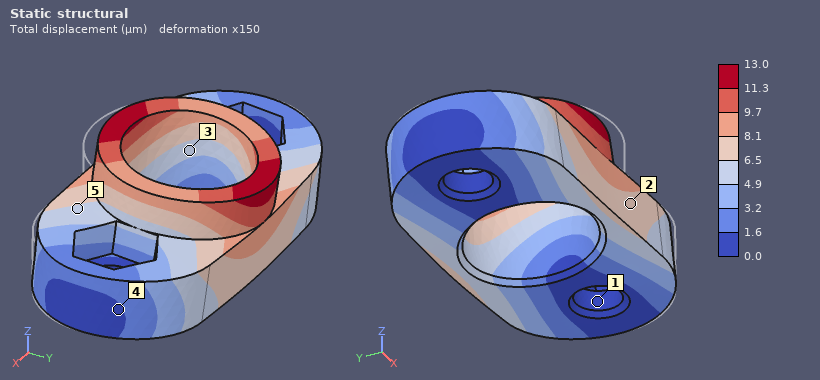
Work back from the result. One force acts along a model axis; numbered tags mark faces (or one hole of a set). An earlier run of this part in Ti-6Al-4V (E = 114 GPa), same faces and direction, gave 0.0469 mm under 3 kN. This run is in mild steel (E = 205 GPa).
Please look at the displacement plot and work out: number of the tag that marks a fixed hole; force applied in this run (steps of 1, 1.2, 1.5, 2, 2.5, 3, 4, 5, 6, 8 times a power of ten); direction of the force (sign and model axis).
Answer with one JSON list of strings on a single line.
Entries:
["1", "1.5 kN", "+Y"]
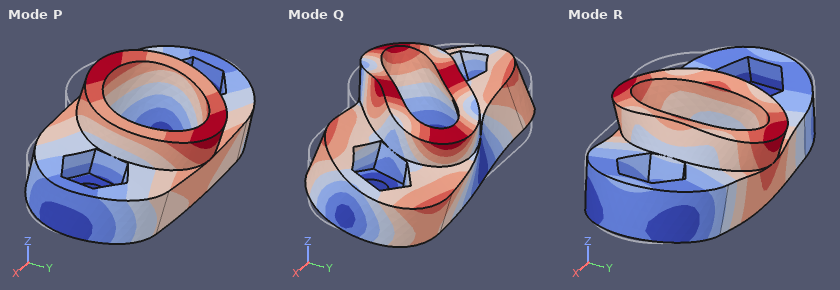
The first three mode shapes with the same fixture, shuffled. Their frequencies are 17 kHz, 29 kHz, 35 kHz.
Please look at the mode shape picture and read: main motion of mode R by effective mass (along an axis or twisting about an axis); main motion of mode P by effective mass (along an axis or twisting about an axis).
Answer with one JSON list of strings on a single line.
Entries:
["along Z", "along Y"]
